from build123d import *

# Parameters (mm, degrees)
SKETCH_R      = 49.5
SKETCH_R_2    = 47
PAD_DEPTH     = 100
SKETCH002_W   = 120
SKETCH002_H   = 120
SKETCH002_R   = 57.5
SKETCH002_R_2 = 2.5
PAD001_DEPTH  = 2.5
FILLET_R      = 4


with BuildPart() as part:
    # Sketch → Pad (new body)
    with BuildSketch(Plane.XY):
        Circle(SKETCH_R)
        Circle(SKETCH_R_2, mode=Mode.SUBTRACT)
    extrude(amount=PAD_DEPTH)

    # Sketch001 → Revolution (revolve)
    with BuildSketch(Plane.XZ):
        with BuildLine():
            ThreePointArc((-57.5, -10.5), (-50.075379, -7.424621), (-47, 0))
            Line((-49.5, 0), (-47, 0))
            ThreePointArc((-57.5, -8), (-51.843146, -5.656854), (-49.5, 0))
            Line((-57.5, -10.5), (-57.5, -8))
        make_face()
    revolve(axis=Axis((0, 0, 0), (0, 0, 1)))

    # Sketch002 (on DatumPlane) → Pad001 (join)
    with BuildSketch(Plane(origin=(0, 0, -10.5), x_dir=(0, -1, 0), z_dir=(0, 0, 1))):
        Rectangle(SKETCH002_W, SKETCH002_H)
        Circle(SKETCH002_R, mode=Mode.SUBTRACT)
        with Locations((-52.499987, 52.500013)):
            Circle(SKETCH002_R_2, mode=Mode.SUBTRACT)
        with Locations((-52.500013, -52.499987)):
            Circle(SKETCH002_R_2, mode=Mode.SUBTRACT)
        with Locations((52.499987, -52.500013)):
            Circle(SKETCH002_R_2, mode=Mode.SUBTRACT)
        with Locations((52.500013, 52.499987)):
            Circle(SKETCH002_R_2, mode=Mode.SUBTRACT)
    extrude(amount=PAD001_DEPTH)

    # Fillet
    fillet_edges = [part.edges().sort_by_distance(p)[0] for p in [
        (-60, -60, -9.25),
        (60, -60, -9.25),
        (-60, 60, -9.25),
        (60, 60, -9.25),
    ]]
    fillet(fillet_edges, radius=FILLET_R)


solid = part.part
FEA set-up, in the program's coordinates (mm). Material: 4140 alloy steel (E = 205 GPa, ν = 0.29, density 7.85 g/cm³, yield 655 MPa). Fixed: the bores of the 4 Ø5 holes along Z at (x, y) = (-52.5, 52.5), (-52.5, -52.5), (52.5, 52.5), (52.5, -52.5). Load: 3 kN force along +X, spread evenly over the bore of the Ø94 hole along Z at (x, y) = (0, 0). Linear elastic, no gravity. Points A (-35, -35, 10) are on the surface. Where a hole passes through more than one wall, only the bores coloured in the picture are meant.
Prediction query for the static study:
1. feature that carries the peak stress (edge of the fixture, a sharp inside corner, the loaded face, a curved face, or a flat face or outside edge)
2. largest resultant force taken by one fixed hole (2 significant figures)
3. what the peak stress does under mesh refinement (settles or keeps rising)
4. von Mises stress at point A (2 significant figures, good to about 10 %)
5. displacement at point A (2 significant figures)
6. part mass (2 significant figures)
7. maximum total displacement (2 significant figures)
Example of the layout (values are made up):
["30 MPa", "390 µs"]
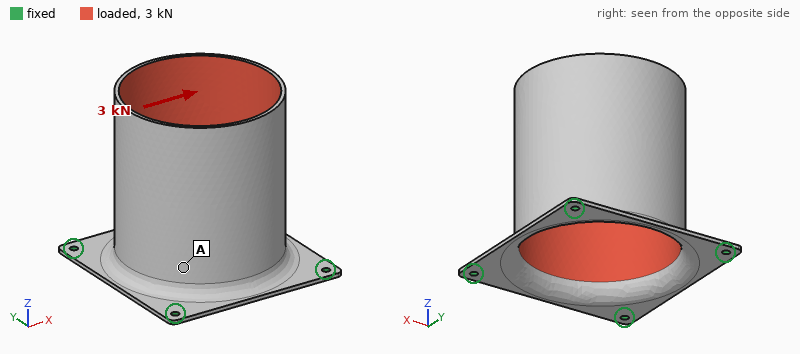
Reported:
["edge of the fixture", "1.5 kN", "keeps rising", "41 MPa", "0.16 mm", "760 g", "0.48 mm"]
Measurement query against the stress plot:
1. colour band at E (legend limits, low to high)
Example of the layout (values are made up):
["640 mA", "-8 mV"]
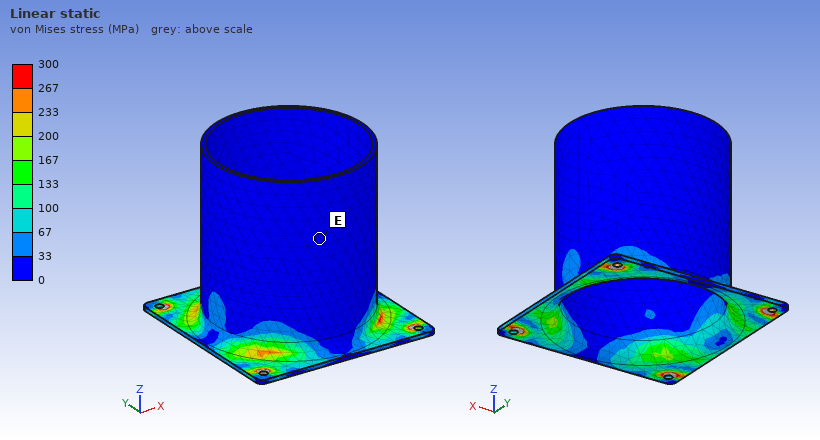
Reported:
["0 to 33 MPa"]
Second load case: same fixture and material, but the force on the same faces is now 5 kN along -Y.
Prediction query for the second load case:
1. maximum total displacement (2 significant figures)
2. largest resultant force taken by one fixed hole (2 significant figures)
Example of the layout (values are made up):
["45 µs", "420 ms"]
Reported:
["0.81 mm", "2.5 kN"]
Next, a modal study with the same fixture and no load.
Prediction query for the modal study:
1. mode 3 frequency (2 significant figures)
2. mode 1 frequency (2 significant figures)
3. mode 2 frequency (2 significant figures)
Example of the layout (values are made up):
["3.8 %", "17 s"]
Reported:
["790 Hz", "570 Hz", "570 Hz"]
